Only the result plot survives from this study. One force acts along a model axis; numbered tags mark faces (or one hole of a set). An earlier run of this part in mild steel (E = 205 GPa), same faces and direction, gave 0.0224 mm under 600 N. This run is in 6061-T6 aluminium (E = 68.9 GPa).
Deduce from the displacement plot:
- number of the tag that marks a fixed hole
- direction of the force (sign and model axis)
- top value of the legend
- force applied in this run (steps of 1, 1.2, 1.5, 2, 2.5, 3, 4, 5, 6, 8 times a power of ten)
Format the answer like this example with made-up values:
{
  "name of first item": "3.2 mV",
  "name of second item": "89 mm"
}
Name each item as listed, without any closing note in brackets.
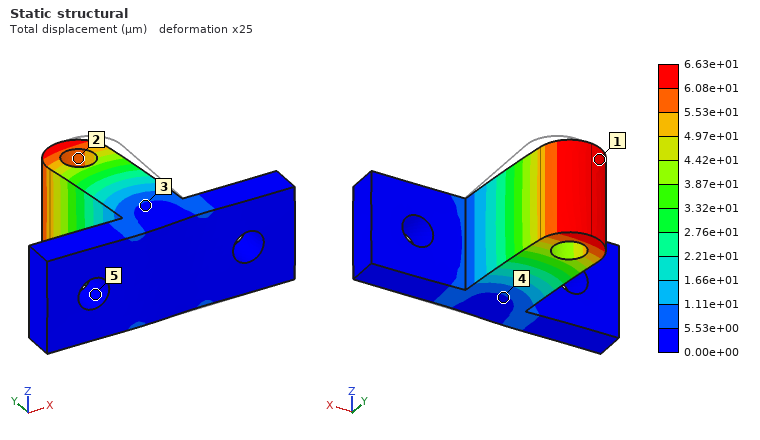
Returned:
{
  "number of the tag that marks a fixed hole": "5",
  "direction of the force": "-X",
  "top value of the legend": "6.63e+01 µm",
  "force applied in this run": "600 N"
}
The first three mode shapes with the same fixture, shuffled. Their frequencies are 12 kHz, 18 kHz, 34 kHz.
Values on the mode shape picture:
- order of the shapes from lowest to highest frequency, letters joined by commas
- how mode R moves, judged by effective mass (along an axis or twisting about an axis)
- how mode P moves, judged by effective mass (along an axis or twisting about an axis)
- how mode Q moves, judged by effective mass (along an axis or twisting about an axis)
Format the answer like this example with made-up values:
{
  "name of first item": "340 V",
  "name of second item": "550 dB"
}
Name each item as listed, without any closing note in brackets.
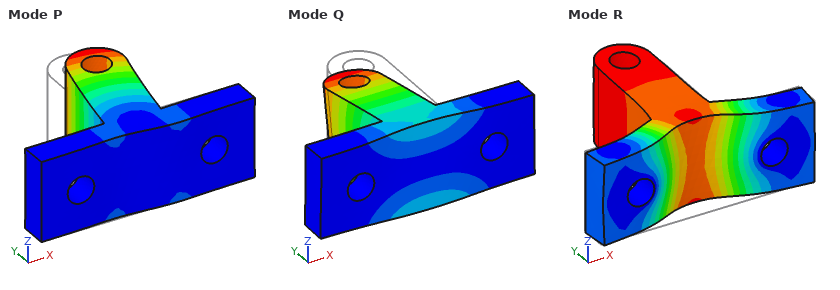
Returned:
{
  "order of the shapes from lowest to highest frequency, letters joined by commas": "Q, P, R",
  "how mode R moves, judged by effective mass": "along Y",
  "how mode P moves, judged by effective mass": "along X",
  "how mode Q moves, judged by effective mass": "along Z"
}
